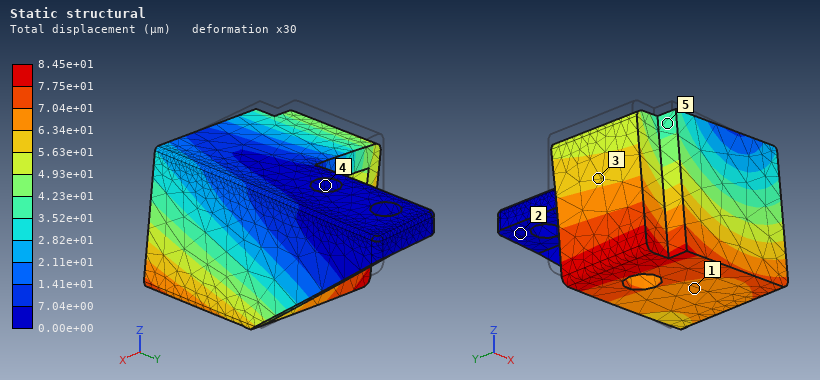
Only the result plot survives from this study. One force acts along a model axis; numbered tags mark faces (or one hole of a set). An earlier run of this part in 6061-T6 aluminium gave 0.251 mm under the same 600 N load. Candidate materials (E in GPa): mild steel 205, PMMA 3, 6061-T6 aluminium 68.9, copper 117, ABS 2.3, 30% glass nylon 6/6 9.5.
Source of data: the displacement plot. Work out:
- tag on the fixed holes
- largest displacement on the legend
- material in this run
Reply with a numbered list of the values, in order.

1. 4
2. 8.45e+01 µm
3. mild steel
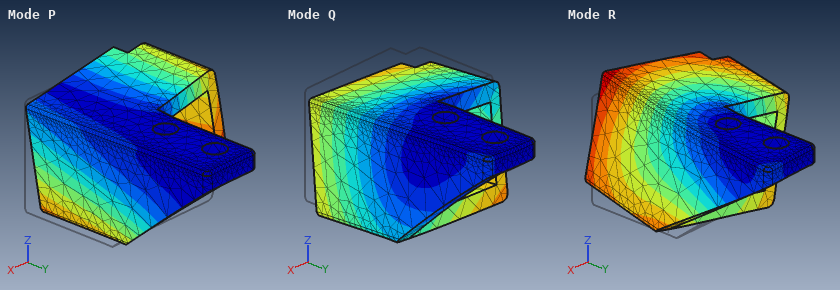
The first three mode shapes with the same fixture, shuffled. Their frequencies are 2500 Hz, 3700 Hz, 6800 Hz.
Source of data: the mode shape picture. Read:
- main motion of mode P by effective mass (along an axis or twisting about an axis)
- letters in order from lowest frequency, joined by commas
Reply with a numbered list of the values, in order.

1. along X
2. P, Q, R
